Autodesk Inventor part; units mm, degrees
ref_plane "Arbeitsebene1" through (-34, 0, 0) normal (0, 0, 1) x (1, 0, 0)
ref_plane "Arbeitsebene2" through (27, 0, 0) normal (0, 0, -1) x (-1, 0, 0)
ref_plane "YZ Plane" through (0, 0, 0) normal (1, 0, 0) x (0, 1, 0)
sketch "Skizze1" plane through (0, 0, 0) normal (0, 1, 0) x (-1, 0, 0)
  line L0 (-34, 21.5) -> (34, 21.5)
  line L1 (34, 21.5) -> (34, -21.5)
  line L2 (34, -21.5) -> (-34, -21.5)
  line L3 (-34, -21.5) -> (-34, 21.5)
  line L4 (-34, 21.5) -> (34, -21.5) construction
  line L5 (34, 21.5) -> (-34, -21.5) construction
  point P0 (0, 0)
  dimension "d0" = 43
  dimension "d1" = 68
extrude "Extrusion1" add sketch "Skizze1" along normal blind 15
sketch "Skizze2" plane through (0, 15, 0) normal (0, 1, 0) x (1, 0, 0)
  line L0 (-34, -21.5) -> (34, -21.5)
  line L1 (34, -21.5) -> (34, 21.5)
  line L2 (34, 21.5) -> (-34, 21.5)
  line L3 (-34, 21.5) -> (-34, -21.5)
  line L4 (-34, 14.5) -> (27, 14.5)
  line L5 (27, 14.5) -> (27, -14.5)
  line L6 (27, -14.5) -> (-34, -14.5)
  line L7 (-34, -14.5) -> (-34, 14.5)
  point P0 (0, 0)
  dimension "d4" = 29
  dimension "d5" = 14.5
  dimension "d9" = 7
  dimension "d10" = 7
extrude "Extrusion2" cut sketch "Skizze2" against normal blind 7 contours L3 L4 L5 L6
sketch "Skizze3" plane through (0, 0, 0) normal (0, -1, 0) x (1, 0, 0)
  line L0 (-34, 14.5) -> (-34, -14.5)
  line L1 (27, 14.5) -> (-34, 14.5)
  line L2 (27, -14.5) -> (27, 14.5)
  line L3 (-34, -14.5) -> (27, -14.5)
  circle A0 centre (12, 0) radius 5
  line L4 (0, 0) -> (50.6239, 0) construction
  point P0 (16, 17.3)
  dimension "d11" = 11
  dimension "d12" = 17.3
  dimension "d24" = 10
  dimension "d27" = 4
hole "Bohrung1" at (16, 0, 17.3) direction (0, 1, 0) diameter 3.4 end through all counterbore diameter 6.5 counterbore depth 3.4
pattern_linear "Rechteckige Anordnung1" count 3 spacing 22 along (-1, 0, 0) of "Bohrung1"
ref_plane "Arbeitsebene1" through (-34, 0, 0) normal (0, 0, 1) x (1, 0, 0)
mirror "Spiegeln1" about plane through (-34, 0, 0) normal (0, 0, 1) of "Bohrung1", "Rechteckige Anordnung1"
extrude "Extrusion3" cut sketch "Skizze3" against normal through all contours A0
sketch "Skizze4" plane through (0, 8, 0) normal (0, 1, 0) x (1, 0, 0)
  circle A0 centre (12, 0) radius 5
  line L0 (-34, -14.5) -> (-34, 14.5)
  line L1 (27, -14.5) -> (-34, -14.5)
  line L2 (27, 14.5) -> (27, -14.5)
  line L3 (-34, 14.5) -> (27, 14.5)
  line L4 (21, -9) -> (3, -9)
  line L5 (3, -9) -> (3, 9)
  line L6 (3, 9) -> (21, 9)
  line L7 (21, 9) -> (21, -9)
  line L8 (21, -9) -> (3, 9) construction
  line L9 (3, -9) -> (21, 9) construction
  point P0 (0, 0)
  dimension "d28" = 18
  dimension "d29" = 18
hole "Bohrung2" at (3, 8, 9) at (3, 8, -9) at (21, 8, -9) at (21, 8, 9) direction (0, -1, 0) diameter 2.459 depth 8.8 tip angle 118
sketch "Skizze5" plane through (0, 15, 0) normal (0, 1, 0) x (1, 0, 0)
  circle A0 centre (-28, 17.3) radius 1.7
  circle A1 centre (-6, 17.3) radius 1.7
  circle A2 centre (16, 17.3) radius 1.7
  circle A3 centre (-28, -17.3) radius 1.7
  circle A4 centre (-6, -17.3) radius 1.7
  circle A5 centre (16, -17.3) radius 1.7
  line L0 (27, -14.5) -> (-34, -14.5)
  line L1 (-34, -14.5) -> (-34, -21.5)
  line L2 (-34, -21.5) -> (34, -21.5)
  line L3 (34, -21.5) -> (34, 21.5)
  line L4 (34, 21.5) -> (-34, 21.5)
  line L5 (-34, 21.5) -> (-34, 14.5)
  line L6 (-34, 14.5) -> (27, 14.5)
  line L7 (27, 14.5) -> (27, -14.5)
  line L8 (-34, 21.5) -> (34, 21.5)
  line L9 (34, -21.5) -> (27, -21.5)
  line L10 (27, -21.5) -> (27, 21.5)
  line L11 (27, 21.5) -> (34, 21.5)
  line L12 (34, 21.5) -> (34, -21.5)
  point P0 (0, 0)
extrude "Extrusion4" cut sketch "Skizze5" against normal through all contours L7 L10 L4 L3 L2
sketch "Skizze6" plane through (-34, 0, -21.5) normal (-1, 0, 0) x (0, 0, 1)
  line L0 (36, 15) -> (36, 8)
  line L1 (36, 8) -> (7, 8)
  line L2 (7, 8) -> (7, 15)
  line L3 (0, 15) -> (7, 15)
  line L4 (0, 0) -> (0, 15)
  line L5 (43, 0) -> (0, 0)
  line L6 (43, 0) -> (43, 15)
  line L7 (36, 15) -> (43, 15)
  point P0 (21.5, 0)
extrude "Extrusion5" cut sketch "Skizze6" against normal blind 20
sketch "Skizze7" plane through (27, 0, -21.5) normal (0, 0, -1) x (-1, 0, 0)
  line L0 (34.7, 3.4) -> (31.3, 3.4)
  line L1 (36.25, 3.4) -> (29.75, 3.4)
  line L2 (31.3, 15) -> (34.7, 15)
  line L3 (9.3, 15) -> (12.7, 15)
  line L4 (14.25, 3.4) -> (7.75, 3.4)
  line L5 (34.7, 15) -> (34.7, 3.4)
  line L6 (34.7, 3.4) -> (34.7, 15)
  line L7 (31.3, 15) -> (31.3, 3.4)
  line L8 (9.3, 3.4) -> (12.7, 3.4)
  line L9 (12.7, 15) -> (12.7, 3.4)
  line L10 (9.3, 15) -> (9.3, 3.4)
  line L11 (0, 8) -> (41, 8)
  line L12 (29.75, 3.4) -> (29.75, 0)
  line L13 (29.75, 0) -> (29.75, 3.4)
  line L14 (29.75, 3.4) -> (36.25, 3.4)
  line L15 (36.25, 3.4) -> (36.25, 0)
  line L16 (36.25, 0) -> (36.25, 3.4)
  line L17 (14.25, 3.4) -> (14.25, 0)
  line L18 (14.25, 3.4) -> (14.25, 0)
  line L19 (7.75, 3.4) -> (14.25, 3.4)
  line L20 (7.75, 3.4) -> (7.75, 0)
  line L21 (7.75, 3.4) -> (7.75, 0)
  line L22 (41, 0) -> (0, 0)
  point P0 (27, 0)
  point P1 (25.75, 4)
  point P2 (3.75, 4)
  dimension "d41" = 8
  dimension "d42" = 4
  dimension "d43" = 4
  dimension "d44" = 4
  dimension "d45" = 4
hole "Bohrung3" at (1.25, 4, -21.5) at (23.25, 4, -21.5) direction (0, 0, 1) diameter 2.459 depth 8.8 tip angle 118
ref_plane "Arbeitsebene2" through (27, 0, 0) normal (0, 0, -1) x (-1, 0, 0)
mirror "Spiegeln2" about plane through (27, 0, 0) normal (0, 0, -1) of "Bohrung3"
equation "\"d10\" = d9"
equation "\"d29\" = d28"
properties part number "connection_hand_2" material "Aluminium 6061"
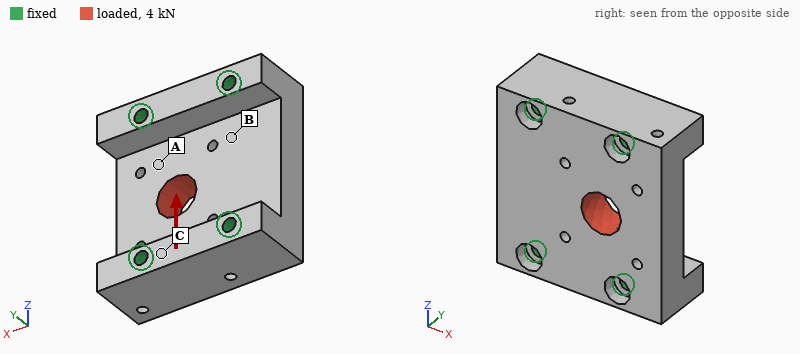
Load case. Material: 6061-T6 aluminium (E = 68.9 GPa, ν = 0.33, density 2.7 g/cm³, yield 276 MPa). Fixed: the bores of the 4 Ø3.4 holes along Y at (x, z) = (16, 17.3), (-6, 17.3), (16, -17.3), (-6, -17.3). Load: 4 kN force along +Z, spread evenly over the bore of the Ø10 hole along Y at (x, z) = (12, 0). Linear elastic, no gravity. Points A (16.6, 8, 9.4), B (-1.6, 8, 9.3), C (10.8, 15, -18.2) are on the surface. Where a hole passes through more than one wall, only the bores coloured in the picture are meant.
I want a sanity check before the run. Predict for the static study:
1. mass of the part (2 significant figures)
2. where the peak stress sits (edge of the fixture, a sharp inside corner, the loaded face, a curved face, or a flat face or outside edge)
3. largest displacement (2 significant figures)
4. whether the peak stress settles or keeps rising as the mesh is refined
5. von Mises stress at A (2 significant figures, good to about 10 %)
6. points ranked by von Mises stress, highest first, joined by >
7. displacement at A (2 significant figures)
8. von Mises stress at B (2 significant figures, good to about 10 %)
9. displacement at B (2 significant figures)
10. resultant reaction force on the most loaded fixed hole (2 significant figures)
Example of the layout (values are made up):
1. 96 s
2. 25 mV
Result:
1. 44 g
2. edge of the fixture
3. 4.6 µm
4. keeps rising
5. 22 MPa
6. A > B > C
7. 2.3 µm
8. 11 MPa
9. 1.3 µm
10. 1.4 kN
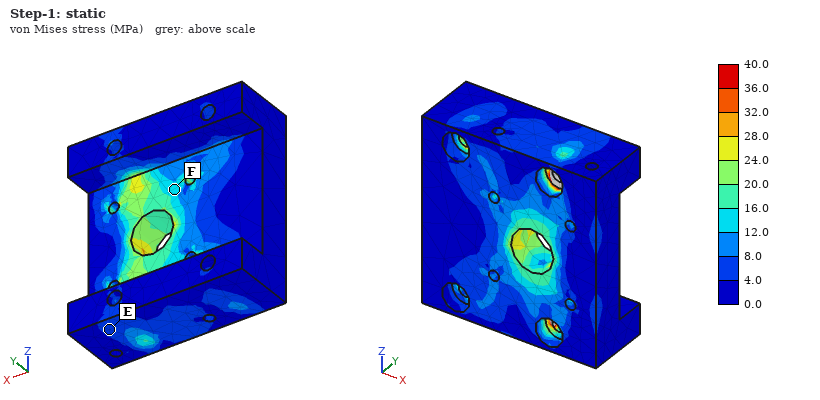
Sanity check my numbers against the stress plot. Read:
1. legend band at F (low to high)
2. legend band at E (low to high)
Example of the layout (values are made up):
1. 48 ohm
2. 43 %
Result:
1. 12.0 to 16.0 MPa
2. 4.0 to 8.0 MPa
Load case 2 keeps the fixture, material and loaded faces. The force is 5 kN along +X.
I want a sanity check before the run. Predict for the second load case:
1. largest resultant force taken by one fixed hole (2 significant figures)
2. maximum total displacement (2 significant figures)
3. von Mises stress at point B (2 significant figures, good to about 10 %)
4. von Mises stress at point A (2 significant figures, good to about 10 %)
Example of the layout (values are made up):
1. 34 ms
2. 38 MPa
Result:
1. 1.4 kN
2. 10 µm
3. 19 MPa
4. 19 MPa
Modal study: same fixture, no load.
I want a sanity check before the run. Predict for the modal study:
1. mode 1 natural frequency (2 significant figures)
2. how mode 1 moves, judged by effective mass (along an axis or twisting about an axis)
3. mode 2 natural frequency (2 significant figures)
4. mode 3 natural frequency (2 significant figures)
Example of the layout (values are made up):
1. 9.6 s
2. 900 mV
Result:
1. 22 kHz
2. along Y
3. 25 kHz
4. 35 kHz
